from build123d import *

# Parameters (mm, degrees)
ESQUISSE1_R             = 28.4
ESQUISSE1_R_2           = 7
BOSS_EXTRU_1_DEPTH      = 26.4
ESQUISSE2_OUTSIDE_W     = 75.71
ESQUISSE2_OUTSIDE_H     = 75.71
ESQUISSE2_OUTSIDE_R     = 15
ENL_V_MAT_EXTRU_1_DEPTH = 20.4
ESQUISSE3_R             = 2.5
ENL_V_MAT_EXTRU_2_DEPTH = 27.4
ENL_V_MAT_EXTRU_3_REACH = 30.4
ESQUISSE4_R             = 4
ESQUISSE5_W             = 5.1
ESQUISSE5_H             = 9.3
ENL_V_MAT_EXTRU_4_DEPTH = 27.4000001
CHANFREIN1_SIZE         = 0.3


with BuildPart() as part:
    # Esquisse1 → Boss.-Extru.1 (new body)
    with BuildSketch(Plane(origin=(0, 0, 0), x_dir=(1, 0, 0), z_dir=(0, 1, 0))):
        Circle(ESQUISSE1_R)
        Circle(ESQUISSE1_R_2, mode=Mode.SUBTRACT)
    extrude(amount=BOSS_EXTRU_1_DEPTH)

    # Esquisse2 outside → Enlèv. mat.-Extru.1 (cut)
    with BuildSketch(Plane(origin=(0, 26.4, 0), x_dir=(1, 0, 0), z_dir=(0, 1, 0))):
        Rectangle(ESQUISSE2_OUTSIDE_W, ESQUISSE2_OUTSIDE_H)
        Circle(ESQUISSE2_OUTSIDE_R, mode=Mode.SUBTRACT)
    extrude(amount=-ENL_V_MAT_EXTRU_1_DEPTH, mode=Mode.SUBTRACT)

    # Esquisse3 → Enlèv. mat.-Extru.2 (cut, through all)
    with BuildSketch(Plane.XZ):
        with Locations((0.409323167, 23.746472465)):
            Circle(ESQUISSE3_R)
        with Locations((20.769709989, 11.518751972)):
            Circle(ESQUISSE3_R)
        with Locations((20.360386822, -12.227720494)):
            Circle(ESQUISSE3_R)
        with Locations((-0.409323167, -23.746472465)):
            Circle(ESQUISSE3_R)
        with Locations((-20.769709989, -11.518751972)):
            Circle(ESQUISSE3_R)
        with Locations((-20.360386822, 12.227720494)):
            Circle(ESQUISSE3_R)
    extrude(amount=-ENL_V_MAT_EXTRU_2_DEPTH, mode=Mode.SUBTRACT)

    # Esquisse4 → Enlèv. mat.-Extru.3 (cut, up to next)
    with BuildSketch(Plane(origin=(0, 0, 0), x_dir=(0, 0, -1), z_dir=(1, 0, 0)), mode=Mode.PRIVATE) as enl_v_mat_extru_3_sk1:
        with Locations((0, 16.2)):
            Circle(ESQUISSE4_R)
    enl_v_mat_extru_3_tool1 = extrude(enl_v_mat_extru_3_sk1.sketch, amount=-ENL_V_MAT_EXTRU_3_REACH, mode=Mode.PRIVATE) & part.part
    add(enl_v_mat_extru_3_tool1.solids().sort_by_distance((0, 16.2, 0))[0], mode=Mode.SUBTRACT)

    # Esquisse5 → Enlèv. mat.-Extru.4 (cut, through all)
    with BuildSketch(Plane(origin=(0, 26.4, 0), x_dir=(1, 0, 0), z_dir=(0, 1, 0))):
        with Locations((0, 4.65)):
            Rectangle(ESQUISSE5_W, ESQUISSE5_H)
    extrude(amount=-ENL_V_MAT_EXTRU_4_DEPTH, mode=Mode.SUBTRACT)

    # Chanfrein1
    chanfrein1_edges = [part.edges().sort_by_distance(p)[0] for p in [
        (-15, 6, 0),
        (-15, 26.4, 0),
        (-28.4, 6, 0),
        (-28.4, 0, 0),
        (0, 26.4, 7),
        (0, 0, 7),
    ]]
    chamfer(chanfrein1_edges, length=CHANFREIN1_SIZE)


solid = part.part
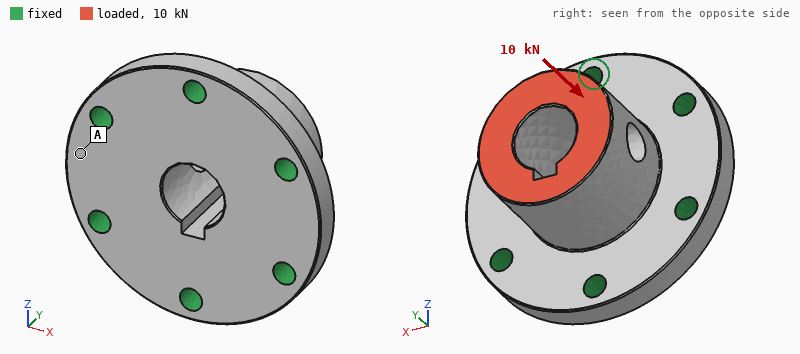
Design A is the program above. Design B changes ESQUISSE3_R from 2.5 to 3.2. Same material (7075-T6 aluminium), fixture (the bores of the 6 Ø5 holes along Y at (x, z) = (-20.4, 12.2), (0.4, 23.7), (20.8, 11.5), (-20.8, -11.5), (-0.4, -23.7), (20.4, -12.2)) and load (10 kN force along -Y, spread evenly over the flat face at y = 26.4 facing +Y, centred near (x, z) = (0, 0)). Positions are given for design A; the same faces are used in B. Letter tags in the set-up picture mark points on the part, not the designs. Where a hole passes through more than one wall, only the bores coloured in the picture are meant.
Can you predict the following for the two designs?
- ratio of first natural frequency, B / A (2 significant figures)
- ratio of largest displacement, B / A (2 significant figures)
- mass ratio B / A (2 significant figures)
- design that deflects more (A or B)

1.0
0.89
0.98
A
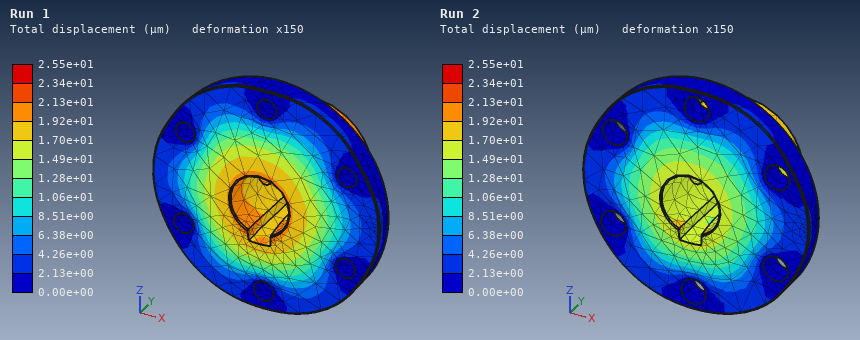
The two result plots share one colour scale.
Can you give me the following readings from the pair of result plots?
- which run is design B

Run 2
